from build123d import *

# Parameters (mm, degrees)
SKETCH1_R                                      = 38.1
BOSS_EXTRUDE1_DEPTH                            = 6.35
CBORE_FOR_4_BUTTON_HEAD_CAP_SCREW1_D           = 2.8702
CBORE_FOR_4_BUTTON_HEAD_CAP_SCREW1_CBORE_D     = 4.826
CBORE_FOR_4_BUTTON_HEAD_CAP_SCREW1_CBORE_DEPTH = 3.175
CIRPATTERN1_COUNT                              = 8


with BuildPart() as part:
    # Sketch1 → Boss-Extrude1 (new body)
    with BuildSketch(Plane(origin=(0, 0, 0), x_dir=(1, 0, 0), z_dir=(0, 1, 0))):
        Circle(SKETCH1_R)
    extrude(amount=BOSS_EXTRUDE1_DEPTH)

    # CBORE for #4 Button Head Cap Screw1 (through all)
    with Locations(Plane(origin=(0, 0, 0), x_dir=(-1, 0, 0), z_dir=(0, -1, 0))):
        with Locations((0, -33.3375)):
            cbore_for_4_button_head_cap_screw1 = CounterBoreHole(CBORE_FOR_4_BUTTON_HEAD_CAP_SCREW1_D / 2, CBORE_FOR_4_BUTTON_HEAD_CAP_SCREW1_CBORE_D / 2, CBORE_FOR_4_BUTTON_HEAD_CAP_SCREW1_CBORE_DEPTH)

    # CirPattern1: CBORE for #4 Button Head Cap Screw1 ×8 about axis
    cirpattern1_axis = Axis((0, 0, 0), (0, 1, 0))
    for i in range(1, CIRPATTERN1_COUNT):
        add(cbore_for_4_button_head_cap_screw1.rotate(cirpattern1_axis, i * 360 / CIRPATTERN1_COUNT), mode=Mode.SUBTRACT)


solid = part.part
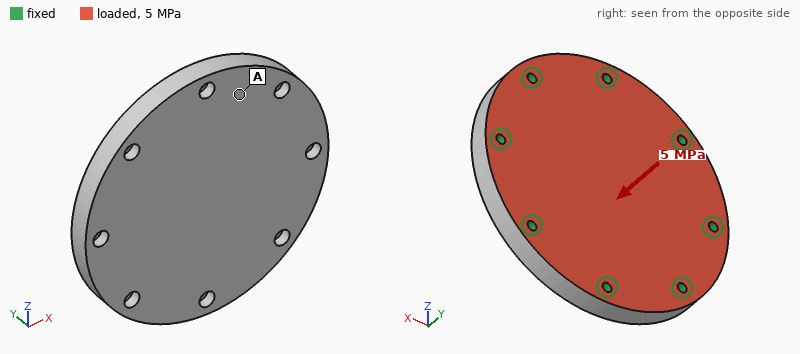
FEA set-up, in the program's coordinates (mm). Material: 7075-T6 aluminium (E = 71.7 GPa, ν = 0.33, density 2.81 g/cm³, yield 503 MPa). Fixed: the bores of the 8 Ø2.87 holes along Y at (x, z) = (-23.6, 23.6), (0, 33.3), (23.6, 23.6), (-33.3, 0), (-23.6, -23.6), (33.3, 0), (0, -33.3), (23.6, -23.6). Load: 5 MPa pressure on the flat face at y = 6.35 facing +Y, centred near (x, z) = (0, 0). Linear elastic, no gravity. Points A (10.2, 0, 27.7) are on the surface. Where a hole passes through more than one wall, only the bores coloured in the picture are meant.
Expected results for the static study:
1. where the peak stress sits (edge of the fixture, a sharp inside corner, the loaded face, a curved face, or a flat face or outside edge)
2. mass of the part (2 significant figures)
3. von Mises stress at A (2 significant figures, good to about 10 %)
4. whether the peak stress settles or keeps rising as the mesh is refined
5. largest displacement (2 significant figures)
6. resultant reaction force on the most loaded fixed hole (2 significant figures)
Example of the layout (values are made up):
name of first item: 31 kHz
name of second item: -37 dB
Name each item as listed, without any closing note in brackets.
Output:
where the peak stress sits: edge of the fixture
mass of the part: 80 g
von Mises stress at A: 68 MPa
whether the peak stress settles or keeps rising as the mesh is refined: keeps rising
largest displacement: 0.13 mm
resultant reaction force on the most loaded fixed hole: 3.3 kN
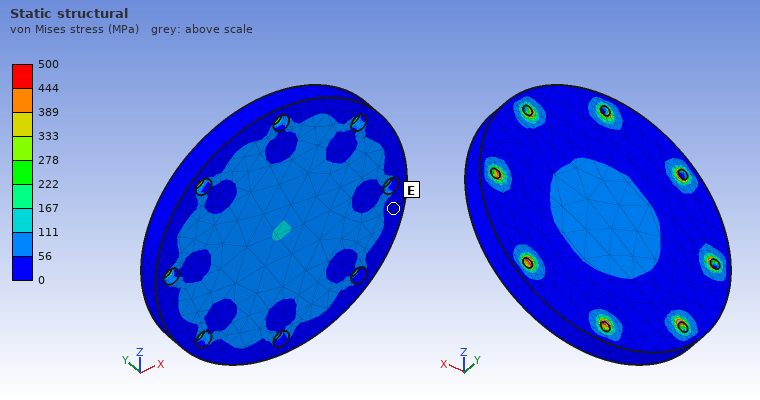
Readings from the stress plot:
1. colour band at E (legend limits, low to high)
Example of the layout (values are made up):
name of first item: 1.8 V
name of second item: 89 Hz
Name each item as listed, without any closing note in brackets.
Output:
colour band at E: 0 to 56 MPa
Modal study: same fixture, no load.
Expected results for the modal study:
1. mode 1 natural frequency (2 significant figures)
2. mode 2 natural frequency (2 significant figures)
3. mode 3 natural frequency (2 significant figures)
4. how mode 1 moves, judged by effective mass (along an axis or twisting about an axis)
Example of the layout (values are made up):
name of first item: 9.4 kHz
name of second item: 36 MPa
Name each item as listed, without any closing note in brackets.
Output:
mode 1 natural frequency: 9100 Hz
mode 2 natural frequency: 19 kHz
mode 3 natural frequency: 19 kHz
how mode 1 moves, judged by effective mass: along Y
